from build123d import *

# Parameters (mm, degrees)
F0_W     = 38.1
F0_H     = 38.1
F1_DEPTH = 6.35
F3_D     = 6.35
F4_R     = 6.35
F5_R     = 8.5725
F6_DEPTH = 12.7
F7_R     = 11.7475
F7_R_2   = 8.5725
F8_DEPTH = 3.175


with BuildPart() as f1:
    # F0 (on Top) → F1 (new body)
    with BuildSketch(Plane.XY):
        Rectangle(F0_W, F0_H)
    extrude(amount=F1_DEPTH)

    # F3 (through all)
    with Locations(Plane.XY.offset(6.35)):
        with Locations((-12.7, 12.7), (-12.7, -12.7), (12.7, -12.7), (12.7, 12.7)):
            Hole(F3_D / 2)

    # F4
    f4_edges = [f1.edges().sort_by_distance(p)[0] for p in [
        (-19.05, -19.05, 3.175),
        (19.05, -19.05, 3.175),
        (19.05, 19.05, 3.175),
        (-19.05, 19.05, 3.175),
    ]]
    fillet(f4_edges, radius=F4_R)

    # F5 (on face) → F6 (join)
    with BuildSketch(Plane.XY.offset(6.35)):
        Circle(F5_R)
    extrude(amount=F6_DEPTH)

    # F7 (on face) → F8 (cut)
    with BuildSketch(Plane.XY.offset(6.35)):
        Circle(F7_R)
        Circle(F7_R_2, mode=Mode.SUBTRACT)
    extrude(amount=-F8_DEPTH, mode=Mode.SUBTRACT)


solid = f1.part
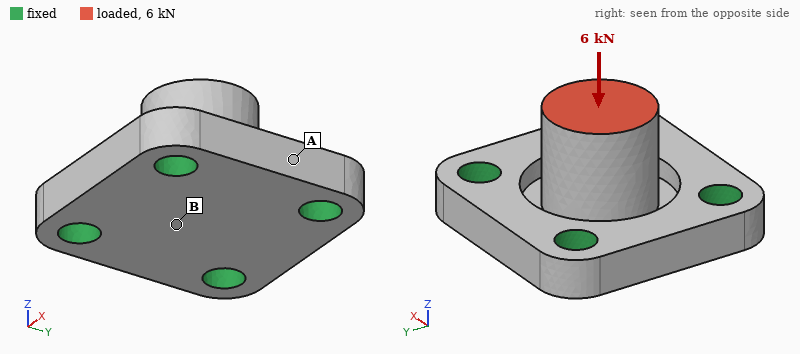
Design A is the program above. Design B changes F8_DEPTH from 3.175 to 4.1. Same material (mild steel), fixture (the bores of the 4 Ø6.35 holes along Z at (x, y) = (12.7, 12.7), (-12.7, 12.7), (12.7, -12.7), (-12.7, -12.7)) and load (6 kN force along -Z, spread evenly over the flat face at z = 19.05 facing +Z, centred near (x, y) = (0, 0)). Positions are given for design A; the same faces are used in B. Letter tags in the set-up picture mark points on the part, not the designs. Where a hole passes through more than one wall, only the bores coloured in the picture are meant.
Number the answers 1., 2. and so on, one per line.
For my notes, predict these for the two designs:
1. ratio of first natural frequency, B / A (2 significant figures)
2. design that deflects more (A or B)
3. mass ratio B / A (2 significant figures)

1. 0.79
2. B
3. 0.98
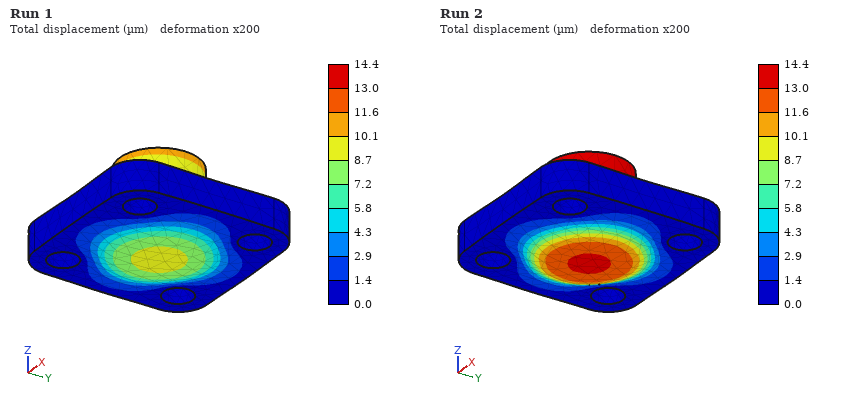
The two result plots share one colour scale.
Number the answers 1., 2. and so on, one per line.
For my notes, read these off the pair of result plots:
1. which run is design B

1. Run 2
